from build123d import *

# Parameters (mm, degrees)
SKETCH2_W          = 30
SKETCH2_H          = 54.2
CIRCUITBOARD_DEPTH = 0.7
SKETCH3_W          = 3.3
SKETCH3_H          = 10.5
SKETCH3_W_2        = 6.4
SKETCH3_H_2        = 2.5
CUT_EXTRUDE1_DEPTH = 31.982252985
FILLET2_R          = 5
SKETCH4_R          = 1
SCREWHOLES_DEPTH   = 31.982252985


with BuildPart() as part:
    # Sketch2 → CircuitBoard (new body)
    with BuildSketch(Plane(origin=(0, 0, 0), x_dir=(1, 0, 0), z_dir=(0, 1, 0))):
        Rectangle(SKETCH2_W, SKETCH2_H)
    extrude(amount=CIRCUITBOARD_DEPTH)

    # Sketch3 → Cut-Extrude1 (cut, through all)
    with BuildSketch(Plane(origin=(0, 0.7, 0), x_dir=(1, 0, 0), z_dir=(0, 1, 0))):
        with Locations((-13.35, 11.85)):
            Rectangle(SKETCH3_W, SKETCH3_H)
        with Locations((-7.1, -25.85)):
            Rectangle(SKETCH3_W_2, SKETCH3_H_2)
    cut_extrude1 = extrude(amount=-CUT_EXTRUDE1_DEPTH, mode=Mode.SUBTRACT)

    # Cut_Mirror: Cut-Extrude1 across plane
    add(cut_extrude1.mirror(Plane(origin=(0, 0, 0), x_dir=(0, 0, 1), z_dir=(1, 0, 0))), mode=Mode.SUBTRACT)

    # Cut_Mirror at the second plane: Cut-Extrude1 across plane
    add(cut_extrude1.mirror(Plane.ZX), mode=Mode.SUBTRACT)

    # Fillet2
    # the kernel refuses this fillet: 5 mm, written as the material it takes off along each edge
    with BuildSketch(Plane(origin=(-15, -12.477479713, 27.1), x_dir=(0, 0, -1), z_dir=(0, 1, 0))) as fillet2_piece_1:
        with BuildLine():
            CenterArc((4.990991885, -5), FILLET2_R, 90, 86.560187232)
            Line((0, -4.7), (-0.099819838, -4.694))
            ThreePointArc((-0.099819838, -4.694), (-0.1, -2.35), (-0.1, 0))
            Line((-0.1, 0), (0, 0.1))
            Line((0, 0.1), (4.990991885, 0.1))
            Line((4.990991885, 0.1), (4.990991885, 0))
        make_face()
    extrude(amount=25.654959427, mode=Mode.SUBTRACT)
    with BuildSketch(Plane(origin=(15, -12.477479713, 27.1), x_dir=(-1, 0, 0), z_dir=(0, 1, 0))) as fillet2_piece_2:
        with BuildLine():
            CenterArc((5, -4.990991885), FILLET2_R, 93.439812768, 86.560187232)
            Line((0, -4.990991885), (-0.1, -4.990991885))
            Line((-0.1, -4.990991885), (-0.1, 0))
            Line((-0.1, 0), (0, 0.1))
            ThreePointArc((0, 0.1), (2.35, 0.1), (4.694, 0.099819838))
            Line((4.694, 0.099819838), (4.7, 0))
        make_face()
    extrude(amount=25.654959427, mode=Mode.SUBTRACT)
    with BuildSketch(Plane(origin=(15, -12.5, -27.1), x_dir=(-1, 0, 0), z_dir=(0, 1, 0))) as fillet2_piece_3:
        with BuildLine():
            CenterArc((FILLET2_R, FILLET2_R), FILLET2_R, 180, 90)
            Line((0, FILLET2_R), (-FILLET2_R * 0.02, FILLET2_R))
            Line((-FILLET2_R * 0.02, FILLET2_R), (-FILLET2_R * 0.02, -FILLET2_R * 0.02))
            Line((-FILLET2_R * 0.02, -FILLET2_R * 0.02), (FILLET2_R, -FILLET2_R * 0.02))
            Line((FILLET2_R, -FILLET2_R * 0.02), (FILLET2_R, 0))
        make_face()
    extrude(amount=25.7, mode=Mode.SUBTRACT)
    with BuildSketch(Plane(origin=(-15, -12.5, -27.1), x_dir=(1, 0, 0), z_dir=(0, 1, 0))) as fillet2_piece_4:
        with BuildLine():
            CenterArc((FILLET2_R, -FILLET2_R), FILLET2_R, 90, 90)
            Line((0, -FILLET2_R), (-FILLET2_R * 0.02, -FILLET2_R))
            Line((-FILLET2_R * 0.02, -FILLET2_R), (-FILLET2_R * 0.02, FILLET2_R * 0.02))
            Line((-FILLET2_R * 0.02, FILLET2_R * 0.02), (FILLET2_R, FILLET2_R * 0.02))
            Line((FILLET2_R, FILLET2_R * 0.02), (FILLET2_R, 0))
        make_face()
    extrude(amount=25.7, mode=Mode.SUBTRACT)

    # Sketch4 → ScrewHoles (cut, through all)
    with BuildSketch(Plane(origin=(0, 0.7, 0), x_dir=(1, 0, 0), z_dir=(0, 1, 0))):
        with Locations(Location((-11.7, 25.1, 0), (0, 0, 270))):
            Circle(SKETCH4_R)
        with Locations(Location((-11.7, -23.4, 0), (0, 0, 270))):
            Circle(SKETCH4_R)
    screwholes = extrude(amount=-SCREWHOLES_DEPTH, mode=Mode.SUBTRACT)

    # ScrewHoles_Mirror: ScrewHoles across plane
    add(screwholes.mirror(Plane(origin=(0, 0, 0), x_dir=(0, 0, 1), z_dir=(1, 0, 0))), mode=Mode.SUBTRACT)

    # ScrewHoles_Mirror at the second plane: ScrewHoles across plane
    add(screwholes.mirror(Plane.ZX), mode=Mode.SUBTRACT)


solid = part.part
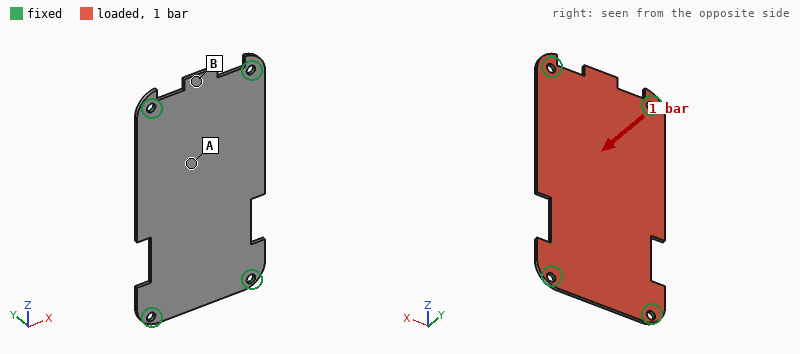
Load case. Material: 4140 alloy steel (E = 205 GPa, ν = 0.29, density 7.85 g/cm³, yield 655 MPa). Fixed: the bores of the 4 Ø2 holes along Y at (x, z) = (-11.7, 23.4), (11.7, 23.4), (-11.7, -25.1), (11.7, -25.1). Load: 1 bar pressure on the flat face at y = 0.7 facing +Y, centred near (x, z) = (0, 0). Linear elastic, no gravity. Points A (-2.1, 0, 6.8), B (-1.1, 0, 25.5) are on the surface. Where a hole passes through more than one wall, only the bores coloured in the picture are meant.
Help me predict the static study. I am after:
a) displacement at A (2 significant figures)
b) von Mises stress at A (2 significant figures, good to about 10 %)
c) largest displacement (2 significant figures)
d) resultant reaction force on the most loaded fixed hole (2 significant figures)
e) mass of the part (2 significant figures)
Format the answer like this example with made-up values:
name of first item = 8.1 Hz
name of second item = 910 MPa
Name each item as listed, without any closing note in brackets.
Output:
displacement at A = 0.24 mm
von Mises stress at A = 81 MPa
largest displacement = 0.30 mm
resultant reaction force on the most loaded fixed hole = 39 N
mass of the part = 8.2 g
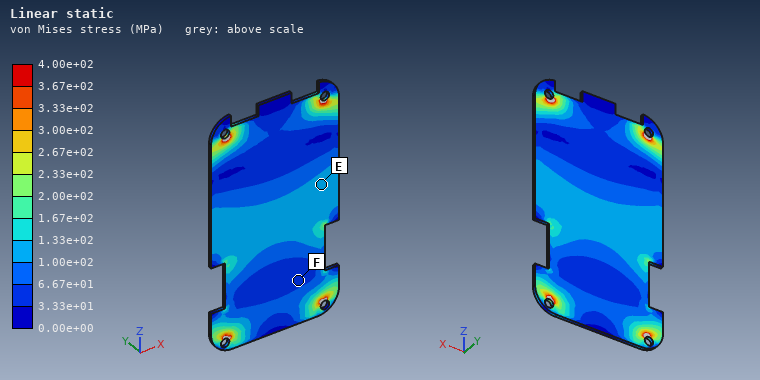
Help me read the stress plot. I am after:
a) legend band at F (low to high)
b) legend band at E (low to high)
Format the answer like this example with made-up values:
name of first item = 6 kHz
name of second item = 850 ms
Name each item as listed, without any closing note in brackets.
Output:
legend band at F = 3.33e+01 to 6.67e+01 MPa
legend band at E = 1.00e+02 to 1.33e+02 MPa
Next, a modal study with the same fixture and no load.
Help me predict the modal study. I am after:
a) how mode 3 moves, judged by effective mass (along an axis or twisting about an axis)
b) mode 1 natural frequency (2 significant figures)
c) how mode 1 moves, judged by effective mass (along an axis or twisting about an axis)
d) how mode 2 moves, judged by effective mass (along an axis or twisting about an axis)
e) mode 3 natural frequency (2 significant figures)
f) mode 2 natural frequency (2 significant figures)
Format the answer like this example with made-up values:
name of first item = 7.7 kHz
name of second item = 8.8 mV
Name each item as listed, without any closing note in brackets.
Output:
how mode 3 moves, judged by effective mass = twisting about X
mode 1 natural frequency = 1400 Hz
how mode 1 moves, judged by effective mass = along Y
how mode 2 moves, judged by effective mass = twisting about Z
mode 3 natural frequency = 3900 Hz
mode 2 natural frequency = 2400 Hz
